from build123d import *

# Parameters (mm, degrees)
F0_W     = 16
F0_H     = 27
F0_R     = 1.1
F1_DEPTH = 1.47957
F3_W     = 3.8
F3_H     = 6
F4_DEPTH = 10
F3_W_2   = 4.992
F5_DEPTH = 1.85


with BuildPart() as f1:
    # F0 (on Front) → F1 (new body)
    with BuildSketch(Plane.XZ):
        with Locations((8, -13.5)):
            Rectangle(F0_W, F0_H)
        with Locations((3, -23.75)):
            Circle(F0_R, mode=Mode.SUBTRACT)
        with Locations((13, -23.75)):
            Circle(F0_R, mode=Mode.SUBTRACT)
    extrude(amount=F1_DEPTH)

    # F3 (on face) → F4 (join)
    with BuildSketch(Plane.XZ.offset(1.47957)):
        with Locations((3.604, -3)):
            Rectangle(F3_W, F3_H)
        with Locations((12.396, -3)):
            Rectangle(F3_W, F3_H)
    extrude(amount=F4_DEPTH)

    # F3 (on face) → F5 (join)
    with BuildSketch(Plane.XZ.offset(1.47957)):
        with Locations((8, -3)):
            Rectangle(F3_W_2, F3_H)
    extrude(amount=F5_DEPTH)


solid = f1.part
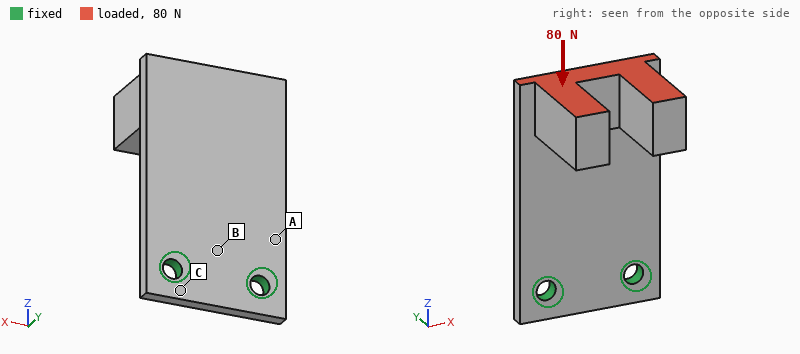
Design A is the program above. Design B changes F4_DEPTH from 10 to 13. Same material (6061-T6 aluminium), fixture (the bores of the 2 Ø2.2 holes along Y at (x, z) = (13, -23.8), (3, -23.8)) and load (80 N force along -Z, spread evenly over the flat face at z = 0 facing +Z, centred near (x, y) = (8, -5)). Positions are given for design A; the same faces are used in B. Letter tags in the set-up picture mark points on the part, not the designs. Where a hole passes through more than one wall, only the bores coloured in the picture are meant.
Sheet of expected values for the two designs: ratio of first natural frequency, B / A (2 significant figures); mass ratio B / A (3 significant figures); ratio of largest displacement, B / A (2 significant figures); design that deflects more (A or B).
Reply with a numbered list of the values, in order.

1. 0.87
2. 1.12
3. 1.5
4. B
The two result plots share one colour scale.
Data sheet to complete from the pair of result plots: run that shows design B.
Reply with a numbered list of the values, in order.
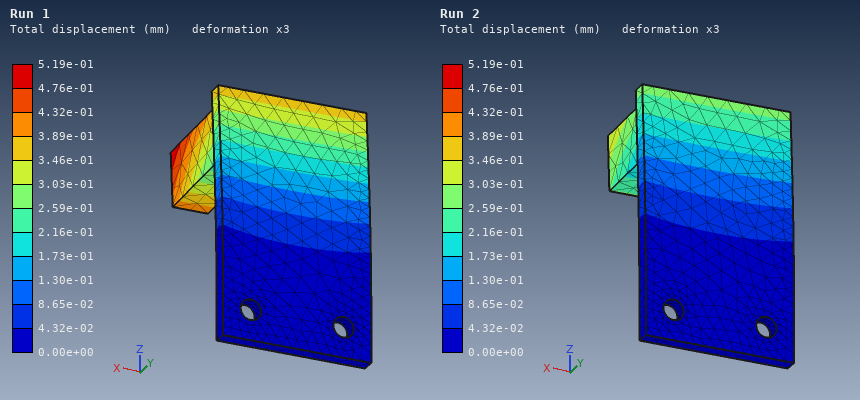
1. Run 1
